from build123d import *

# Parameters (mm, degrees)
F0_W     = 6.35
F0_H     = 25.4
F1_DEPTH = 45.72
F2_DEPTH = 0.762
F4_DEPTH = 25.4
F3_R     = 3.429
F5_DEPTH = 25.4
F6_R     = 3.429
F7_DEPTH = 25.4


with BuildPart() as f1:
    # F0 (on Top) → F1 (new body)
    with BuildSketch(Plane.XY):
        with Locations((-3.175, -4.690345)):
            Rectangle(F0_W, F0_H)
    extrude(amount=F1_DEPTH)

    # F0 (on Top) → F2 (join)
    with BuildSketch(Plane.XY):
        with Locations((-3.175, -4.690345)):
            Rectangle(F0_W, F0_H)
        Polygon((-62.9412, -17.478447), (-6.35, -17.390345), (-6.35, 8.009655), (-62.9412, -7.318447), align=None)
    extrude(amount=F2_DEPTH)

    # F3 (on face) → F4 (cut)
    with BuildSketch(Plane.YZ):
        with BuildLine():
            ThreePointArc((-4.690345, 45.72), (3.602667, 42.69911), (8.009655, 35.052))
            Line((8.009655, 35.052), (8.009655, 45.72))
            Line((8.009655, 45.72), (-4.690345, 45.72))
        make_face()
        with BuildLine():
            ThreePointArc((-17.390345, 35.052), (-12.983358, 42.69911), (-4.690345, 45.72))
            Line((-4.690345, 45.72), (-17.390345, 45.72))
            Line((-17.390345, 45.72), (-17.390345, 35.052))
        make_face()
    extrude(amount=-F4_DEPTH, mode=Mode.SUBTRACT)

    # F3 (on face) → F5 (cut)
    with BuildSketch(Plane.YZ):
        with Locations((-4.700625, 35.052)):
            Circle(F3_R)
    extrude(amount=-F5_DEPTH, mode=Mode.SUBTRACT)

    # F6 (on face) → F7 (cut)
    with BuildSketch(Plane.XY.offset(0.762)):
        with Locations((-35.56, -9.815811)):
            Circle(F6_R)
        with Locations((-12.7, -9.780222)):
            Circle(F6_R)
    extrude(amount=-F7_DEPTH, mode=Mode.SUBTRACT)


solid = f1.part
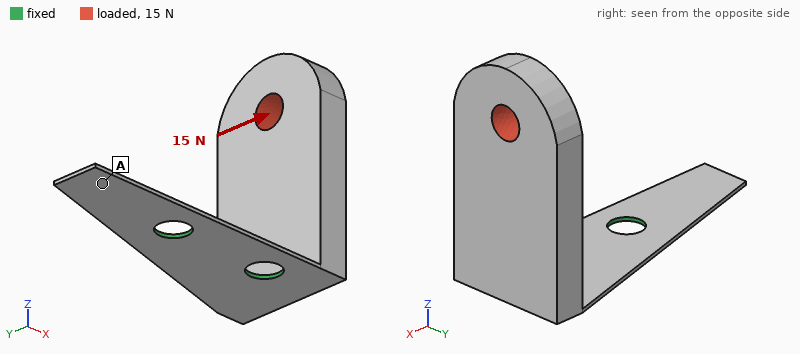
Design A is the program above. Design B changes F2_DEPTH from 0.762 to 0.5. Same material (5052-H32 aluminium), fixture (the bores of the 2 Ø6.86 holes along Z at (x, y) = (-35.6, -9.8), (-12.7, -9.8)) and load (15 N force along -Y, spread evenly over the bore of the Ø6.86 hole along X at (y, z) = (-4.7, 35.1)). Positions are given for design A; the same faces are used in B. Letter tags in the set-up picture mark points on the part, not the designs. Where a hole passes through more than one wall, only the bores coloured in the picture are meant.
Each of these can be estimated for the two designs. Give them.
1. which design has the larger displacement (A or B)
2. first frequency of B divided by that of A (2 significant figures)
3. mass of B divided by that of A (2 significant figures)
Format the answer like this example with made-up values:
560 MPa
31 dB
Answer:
B
0.57
0.97
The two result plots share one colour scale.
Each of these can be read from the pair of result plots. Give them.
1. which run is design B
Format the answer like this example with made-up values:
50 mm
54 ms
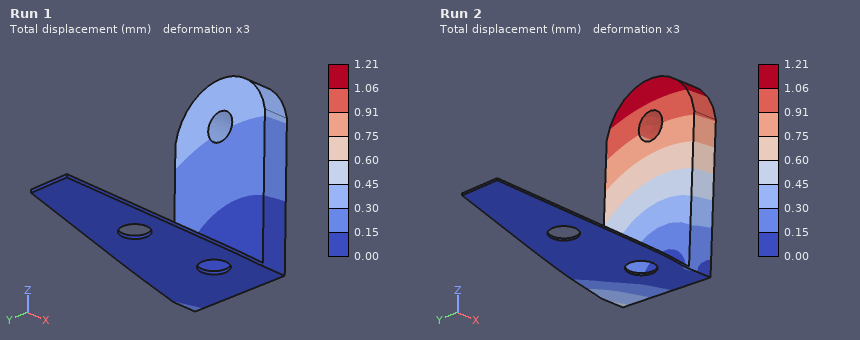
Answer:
Run 2
